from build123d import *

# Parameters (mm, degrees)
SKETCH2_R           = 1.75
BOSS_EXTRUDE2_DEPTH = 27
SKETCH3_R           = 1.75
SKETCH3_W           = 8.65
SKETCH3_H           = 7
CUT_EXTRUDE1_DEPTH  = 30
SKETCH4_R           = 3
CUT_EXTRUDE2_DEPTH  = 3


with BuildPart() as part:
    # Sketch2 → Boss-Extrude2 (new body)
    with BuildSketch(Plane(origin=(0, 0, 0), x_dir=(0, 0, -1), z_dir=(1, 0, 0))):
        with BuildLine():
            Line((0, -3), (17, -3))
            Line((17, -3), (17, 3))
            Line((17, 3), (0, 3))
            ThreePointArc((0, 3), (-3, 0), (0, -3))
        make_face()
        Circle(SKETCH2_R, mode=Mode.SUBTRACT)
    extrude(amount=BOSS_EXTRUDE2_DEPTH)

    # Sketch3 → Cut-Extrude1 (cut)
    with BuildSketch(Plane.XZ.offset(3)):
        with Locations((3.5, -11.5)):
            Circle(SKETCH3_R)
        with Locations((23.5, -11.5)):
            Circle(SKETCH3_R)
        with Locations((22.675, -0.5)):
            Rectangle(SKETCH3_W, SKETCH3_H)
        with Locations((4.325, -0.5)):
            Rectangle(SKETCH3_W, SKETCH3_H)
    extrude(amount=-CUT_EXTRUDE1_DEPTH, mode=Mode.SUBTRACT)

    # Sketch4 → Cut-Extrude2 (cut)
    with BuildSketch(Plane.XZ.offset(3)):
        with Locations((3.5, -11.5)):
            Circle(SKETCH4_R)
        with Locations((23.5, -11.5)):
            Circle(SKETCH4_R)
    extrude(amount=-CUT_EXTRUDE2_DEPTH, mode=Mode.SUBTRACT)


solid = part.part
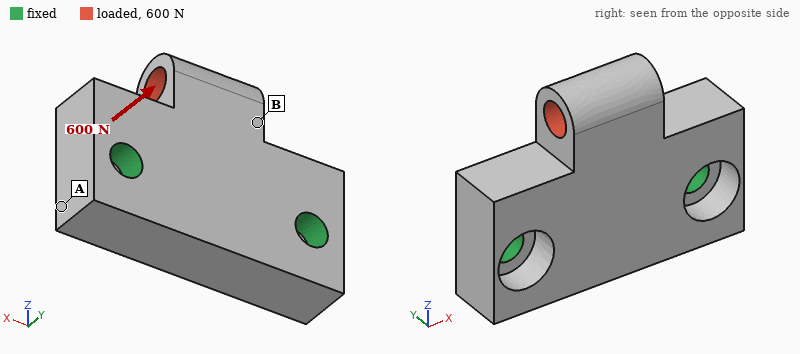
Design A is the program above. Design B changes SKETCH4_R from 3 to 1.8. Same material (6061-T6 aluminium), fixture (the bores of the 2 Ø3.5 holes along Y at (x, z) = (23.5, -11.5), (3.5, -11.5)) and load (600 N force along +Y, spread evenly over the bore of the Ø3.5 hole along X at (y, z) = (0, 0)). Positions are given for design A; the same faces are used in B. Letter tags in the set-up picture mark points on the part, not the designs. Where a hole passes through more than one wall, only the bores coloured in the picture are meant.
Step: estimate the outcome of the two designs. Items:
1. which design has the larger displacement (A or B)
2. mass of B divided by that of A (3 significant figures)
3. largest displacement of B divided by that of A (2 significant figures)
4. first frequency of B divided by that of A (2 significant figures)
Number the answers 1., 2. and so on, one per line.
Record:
1. A
2. 1.05
3. 0.88
4. 1.1
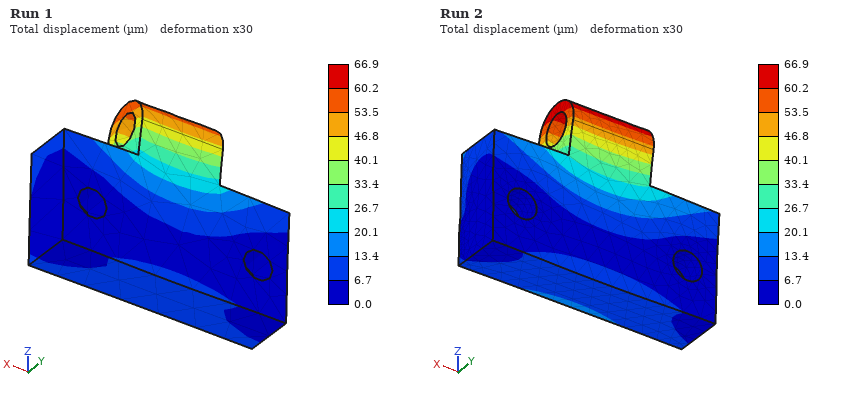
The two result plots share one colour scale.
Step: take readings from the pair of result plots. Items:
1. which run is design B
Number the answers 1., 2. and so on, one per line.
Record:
1. Run 1
